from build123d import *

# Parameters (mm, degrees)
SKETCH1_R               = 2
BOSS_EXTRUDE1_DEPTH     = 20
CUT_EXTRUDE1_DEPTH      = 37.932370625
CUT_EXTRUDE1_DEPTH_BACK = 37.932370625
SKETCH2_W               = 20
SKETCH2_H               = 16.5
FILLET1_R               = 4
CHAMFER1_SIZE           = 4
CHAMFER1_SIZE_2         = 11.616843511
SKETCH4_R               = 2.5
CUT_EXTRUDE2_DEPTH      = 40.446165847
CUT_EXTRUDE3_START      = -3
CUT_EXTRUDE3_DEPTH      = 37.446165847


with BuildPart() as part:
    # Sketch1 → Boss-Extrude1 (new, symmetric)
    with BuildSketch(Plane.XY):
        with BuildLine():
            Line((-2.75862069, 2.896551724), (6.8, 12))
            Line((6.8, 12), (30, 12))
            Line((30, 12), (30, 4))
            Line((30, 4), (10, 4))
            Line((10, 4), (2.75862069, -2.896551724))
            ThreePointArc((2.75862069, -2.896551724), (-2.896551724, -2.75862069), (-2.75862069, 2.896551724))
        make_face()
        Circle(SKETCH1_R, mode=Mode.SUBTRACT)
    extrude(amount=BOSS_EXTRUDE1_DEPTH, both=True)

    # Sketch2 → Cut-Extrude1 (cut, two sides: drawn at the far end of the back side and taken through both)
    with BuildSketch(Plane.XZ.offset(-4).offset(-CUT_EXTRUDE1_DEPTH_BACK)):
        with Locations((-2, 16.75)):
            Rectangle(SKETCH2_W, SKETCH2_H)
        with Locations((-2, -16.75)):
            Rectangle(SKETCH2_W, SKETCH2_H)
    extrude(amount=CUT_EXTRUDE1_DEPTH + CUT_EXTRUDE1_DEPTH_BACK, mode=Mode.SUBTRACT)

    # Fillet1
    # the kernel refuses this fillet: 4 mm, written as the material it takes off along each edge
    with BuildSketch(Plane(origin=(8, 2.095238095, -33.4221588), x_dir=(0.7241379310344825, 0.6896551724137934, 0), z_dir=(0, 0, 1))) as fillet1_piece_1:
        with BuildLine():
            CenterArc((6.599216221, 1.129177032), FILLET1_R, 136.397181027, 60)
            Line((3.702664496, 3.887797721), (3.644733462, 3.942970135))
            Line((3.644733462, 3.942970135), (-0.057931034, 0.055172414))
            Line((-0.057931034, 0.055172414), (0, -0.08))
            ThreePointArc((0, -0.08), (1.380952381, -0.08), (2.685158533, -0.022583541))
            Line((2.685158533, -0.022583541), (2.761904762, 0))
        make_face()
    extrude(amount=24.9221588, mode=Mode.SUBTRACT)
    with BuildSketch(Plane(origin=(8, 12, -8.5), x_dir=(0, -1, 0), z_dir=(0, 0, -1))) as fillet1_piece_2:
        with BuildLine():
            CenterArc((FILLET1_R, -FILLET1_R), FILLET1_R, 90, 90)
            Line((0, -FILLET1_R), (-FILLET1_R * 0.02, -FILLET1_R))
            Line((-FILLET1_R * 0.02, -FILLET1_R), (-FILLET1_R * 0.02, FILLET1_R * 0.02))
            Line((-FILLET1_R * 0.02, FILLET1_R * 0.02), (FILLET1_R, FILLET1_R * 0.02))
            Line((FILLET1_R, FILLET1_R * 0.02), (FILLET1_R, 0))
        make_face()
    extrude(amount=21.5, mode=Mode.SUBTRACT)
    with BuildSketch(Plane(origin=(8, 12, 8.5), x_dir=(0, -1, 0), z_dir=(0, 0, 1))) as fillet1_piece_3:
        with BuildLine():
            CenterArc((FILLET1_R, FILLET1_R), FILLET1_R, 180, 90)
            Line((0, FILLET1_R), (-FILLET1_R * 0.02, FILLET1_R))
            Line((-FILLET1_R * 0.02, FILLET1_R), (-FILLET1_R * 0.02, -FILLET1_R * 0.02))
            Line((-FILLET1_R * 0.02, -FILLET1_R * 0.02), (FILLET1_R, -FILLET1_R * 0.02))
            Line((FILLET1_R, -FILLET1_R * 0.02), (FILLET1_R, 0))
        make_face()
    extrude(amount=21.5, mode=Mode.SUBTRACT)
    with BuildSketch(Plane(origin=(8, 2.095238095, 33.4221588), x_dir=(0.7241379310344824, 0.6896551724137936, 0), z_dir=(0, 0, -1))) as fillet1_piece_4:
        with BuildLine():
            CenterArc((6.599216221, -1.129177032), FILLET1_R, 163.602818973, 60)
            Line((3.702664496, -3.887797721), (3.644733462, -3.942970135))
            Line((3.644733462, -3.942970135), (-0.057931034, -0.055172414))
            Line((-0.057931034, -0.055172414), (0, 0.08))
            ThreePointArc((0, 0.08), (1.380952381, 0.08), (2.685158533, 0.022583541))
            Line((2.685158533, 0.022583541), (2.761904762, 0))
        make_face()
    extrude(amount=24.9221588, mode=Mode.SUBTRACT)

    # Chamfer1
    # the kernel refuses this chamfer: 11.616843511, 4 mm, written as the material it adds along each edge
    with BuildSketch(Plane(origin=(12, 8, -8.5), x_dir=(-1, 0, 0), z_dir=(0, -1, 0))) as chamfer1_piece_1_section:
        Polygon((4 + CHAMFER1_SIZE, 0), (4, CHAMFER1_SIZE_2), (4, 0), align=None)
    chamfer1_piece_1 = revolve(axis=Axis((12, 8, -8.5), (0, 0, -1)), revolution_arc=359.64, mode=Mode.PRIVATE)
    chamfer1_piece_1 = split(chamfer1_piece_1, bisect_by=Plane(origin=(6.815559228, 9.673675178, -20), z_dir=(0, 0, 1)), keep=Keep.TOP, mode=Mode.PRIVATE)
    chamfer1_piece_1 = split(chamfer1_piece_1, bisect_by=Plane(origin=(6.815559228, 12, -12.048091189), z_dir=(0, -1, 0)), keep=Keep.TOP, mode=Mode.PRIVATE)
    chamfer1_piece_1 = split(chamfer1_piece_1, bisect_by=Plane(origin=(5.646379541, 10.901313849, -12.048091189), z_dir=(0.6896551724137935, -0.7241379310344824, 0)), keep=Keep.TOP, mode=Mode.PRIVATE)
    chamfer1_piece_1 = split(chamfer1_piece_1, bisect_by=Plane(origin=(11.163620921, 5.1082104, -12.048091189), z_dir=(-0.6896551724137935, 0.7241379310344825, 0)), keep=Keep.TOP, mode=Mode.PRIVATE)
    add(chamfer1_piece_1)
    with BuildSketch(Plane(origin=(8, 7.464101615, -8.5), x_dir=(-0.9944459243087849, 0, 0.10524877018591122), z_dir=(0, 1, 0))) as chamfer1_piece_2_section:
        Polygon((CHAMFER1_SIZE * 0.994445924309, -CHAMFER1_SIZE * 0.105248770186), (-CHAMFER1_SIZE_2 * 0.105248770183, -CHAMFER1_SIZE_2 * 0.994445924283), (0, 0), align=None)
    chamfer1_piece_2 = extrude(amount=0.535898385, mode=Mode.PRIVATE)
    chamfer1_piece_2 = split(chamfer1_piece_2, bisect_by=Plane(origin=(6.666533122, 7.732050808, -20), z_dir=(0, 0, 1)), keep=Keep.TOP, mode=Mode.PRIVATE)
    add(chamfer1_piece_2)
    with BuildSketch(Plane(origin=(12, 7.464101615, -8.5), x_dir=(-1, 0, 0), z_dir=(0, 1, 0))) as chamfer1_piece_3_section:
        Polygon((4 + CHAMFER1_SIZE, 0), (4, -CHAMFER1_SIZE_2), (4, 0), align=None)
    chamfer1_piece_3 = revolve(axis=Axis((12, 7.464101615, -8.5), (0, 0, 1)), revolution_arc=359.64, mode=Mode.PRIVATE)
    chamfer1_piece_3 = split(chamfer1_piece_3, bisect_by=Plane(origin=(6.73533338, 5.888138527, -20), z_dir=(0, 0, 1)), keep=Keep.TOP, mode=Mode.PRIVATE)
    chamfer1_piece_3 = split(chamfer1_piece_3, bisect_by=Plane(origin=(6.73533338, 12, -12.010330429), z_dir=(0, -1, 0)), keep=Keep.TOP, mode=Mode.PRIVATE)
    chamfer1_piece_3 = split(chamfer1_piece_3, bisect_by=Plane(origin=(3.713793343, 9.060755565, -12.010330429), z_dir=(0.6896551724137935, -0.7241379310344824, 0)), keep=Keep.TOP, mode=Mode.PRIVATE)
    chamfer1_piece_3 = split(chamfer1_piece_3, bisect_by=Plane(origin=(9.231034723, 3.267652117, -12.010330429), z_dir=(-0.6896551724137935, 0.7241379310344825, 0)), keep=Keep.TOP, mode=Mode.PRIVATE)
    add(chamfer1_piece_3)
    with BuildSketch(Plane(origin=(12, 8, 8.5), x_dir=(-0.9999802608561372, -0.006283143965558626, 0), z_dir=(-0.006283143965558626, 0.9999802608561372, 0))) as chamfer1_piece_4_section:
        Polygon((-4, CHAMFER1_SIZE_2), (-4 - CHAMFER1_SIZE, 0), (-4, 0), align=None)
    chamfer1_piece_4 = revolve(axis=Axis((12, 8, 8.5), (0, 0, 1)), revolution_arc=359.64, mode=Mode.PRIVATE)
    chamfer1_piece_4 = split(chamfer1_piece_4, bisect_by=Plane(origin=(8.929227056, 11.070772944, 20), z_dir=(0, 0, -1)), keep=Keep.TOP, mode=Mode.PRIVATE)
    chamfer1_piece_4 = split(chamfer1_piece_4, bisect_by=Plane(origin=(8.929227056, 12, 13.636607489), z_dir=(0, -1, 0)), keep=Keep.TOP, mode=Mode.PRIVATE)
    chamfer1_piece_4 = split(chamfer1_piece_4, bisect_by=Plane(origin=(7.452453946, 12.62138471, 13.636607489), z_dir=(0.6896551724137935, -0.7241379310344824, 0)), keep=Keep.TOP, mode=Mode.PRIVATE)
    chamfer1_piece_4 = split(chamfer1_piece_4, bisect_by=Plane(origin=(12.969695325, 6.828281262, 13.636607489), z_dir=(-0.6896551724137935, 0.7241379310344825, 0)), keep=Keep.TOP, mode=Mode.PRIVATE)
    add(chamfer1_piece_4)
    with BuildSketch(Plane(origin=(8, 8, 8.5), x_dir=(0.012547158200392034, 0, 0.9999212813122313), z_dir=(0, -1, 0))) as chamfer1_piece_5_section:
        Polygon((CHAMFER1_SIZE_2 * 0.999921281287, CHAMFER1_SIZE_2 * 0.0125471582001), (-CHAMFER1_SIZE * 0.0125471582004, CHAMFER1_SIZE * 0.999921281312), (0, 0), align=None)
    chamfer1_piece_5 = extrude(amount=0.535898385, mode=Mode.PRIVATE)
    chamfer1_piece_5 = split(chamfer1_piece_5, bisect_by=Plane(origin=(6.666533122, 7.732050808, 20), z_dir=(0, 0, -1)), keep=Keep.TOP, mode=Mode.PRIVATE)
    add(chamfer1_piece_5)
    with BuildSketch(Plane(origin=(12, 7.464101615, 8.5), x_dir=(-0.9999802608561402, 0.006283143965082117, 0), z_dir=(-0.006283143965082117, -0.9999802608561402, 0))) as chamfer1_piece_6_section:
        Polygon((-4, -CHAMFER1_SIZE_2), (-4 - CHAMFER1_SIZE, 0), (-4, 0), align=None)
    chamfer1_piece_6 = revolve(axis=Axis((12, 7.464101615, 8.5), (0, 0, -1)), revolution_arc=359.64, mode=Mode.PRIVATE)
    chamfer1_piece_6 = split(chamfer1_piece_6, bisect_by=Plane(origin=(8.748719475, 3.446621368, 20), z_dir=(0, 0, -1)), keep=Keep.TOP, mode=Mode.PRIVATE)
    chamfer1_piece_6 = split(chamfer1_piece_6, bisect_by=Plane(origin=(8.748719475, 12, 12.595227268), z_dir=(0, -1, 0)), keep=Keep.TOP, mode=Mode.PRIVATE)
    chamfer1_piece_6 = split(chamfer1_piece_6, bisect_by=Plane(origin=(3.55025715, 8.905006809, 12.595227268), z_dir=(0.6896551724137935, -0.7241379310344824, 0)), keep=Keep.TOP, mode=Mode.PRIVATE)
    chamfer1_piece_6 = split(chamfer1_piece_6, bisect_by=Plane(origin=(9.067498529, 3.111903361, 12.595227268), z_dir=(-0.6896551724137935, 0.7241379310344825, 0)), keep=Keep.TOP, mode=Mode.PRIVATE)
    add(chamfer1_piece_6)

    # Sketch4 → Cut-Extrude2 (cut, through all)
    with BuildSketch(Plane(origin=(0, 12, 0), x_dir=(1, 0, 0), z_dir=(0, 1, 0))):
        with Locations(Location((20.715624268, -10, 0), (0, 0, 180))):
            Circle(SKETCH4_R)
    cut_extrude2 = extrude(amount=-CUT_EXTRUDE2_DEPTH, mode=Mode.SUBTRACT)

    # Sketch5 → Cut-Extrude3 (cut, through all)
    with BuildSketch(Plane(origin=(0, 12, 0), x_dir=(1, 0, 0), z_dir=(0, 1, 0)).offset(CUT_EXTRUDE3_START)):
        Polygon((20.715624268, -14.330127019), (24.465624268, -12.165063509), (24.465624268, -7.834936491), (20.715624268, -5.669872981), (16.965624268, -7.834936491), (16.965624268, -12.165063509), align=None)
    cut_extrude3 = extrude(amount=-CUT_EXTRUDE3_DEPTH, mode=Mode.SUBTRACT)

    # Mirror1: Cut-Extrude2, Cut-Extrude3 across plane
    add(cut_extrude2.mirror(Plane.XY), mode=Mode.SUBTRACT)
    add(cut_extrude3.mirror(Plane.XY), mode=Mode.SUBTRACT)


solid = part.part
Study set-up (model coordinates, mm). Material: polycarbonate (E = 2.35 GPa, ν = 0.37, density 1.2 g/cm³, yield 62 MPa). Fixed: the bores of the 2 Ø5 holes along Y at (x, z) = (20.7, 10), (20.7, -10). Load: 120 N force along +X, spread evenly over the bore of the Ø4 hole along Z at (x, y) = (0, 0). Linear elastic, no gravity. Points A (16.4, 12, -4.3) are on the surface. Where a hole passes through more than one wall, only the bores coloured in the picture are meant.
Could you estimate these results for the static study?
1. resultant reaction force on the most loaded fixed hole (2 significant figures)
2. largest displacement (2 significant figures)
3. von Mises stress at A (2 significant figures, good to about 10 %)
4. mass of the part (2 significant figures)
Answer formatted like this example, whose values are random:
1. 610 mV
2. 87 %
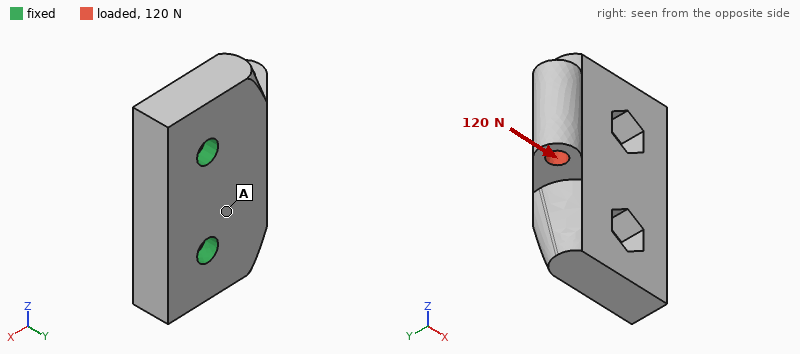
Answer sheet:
1. 60 N
2. 0.27 mm
3. 2.8 MPa
4. 10 g
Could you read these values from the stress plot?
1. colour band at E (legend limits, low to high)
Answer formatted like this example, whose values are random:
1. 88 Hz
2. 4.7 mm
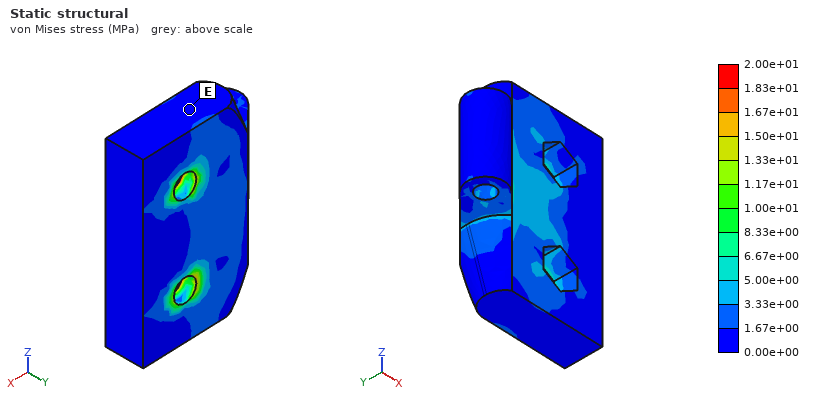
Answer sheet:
1. 0.00e+00 to 1.67e+00 MPa
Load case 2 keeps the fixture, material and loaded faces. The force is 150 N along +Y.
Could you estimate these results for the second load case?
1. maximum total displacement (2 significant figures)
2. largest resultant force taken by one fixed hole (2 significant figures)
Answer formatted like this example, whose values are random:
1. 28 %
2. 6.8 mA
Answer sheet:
1. 0.59 mm
2. 84 N
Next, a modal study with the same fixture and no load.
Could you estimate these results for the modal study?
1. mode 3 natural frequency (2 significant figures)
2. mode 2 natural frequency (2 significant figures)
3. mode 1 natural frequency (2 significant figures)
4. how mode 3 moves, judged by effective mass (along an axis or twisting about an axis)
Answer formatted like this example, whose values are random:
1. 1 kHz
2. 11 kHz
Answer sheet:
1. 5700 Hz
2. 5100 Hz
3. 1900 Hz
4. along Z
